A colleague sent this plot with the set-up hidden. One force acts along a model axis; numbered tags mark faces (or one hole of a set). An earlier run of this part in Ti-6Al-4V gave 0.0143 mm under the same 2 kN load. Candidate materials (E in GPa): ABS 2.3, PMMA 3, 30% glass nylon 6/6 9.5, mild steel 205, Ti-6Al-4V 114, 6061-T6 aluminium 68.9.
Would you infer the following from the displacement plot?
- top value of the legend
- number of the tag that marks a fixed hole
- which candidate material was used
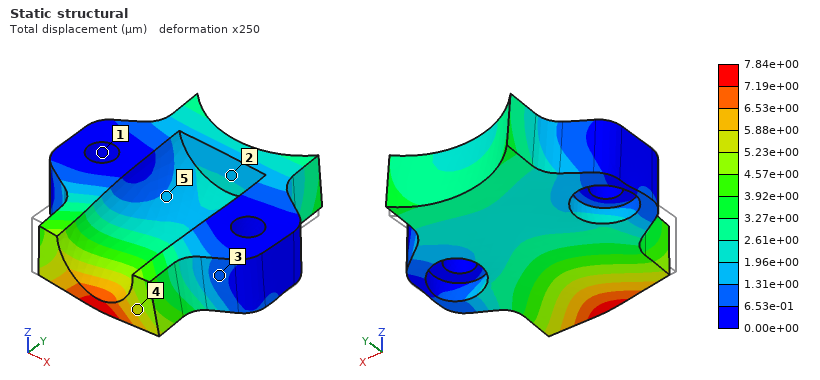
7.84e+00 µm
1
mild steel
